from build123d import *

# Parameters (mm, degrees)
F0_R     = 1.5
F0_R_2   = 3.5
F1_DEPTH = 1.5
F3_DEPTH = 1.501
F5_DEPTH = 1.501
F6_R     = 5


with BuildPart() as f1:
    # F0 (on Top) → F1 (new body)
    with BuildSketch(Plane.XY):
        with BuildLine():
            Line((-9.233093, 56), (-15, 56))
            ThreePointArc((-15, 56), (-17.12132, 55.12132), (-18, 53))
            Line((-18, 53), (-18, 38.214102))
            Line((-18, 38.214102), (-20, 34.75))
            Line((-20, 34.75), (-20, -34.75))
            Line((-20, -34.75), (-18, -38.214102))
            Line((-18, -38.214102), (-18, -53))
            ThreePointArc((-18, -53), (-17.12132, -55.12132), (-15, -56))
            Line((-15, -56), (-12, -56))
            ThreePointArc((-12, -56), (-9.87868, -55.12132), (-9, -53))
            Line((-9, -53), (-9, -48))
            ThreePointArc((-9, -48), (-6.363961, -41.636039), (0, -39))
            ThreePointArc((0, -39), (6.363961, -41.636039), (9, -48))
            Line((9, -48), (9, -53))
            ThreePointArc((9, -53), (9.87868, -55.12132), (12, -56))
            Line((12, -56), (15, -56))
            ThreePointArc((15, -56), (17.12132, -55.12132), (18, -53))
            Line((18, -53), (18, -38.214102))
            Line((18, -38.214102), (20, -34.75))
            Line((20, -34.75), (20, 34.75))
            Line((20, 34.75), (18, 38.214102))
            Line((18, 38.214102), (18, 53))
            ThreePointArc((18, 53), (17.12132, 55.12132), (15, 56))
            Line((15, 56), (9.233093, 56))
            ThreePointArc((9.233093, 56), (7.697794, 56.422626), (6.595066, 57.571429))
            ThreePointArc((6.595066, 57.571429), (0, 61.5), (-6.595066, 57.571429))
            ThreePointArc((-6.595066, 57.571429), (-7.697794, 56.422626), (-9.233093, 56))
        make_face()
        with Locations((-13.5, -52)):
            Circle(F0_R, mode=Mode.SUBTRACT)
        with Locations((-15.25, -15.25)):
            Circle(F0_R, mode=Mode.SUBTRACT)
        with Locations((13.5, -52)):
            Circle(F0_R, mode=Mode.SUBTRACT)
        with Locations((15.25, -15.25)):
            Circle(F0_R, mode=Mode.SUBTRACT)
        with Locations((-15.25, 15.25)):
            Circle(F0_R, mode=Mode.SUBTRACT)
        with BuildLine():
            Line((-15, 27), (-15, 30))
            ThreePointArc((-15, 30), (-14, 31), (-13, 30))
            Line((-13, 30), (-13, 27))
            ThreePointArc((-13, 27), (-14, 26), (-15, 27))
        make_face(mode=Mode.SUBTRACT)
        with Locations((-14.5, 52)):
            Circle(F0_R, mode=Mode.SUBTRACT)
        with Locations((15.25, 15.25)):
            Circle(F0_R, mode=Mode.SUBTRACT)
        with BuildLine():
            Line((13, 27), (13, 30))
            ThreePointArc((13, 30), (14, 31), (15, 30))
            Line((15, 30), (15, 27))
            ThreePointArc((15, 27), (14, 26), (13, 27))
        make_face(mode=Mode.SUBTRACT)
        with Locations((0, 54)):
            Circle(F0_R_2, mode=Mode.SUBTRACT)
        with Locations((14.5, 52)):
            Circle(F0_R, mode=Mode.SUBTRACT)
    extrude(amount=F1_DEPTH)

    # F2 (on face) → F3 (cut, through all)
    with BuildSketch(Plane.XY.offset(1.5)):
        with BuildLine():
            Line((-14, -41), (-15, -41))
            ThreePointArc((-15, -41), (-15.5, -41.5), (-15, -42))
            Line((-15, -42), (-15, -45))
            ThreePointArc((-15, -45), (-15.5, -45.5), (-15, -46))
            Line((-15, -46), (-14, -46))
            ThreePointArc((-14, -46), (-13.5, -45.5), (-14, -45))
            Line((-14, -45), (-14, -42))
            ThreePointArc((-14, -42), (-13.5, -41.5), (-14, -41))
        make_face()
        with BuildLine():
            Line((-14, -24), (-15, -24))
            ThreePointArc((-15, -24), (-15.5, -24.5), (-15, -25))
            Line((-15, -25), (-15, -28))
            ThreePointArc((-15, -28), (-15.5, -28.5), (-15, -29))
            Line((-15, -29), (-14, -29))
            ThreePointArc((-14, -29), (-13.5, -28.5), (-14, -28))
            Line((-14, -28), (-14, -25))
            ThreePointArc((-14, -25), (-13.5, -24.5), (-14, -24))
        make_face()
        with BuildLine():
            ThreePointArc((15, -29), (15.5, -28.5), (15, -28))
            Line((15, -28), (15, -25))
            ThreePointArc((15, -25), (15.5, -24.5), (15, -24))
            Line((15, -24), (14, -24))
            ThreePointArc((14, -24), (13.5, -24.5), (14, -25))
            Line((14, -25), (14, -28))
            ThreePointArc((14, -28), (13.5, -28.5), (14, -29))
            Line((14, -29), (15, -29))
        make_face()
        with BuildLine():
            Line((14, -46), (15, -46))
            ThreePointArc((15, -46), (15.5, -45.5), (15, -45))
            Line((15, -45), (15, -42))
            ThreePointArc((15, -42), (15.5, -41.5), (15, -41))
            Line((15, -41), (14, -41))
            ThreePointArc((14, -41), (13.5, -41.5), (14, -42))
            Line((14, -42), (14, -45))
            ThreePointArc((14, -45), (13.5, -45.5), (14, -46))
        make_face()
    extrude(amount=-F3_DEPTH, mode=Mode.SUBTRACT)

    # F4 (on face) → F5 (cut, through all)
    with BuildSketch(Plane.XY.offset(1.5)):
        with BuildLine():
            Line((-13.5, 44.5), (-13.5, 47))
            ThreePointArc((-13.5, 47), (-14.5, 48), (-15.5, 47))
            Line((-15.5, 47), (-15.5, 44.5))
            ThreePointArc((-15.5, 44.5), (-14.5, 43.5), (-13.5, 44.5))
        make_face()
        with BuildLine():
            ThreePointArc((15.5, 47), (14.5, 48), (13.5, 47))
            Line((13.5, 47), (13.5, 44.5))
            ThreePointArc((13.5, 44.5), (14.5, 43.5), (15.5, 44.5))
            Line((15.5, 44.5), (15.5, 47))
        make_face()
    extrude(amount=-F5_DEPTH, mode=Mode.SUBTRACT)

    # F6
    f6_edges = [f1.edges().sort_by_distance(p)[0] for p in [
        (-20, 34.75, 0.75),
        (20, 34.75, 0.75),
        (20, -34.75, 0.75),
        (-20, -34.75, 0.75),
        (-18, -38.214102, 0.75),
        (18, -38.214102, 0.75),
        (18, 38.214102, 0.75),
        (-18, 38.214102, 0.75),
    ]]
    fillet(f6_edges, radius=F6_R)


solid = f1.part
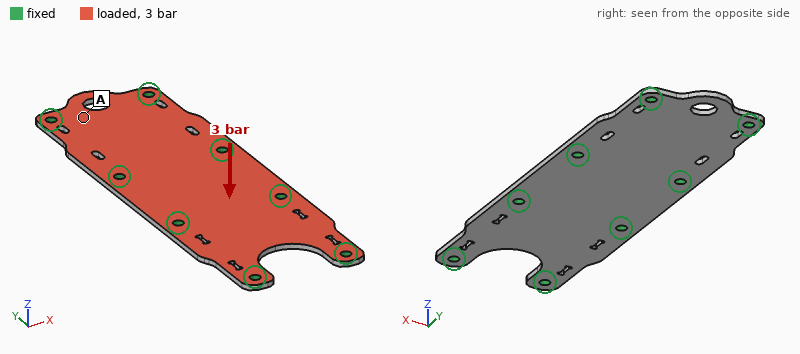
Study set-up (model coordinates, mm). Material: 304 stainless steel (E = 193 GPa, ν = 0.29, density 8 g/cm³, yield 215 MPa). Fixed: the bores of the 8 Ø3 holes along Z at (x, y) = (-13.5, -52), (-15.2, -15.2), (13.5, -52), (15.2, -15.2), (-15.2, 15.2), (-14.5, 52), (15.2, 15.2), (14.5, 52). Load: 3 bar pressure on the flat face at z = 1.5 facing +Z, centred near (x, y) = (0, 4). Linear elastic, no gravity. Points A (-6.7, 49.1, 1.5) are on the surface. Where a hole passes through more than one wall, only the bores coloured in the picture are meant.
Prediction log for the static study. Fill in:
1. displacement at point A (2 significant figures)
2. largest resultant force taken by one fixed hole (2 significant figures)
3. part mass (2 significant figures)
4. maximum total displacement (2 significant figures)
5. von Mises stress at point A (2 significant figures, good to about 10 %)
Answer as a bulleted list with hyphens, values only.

- 13 µm
- 200 N
- 47 g
- 39 µm
- 31 MPa
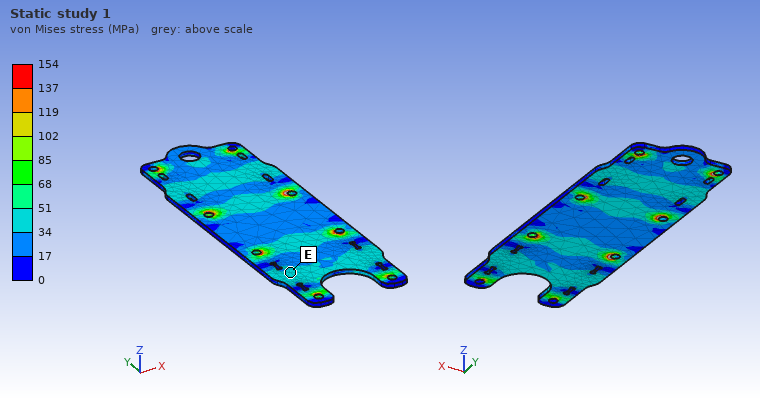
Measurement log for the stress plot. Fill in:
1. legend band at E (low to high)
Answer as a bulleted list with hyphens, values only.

- 34 to 51 MPa
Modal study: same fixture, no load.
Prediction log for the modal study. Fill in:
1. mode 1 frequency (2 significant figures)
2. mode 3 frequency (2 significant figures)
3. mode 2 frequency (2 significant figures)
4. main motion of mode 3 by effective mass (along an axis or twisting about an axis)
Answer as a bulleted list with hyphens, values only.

- 4800 Hz
- 6200 Hz
- 4800 Hz
- along Z
